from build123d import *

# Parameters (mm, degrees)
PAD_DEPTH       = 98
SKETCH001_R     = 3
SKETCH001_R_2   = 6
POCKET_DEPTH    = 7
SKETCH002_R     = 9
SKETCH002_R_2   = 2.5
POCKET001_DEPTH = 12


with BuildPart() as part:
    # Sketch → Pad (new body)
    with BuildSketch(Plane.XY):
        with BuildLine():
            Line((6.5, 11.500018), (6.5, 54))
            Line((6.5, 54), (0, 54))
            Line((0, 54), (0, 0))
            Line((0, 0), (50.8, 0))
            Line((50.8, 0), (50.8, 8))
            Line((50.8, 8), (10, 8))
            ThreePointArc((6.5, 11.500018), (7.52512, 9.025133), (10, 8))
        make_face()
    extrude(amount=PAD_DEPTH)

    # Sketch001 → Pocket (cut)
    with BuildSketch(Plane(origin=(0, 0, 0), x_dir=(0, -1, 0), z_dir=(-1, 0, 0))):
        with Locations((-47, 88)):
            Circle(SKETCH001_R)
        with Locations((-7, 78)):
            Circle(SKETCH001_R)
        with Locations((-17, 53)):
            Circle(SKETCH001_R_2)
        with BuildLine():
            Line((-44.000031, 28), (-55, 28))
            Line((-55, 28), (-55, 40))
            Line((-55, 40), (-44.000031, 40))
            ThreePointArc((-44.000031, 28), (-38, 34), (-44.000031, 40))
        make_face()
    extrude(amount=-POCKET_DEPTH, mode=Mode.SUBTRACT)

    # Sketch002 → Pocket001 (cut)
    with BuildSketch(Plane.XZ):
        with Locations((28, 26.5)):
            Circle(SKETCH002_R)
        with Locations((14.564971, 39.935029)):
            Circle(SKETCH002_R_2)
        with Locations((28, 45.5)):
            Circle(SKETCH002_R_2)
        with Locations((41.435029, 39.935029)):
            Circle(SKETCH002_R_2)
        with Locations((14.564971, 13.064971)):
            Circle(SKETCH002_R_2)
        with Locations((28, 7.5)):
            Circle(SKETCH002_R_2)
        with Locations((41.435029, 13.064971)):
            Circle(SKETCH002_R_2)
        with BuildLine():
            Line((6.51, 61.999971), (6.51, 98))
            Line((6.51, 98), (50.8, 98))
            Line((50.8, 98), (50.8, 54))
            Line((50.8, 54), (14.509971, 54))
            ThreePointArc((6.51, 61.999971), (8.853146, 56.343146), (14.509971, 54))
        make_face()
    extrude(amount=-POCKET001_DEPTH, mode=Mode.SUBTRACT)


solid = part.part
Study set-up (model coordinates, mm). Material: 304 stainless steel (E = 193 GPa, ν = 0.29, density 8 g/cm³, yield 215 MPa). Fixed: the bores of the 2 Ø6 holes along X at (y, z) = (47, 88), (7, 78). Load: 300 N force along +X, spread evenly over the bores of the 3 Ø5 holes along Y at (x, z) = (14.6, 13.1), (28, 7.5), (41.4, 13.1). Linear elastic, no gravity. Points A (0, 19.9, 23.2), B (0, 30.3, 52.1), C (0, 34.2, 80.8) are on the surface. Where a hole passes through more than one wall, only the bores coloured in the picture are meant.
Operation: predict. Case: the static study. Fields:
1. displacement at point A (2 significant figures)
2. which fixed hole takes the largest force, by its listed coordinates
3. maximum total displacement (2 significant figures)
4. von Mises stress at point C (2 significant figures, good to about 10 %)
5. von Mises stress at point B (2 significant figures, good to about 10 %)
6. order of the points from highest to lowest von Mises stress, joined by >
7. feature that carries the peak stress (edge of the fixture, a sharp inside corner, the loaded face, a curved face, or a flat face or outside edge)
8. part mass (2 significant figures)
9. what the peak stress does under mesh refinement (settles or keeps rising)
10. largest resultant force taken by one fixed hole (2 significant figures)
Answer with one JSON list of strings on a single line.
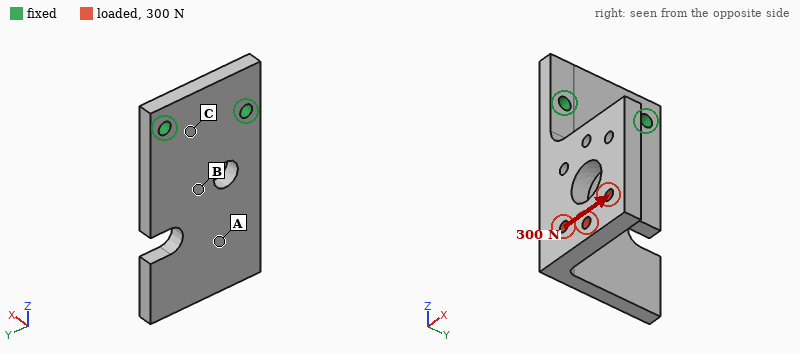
["0.11 mm", "(7, 78)", "0.23 mm", "22 MPa", "38 MPa", "B > C > A", "edge of the fixture", "390 g", "keeps rising", "410 N"]
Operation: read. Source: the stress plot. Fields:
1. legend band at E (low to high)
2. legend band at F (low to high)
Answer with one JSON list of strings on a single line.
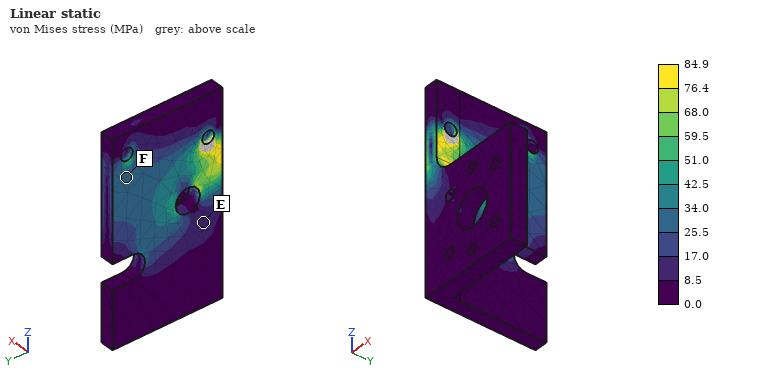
["8.5 to 17.0 MPa", "25.5 to 34.0 MPa"]
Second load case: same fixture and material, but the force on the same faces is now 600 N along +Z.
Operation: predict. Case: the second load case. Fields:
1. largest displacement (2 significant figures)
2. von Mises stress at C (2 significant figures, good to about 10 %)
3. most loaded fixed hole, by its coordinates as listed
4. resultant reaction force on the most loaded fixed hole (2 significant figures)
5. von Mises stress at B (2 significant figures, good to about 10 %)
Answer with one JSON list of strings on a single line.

["0.21 mm", "19 MPa", "(7, 78)", "640 N", "36 MPa"]
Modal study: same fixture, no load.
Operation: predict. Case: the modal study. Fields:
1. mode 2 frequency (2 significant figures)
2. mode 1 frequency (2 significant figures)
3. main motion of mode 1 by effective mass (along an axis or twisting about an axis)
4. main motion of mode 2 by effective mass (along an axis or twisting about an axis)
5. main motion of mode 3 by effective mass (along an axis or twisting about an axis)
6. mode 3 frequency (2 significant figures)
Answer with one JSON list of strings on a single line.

["1100 Hz", "510 Hz", "along X", "along Y", "along Y", "2900 Hz"]
